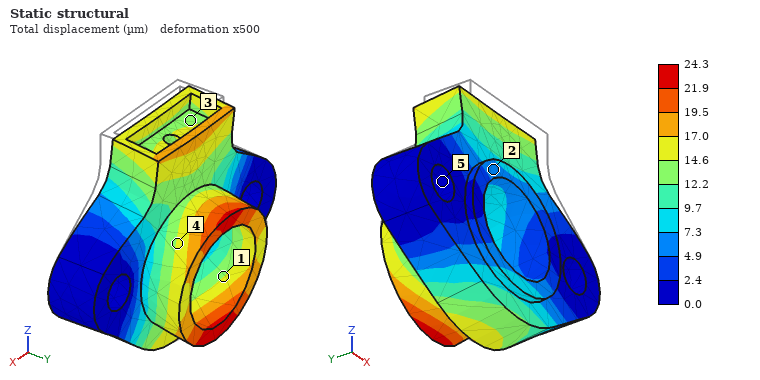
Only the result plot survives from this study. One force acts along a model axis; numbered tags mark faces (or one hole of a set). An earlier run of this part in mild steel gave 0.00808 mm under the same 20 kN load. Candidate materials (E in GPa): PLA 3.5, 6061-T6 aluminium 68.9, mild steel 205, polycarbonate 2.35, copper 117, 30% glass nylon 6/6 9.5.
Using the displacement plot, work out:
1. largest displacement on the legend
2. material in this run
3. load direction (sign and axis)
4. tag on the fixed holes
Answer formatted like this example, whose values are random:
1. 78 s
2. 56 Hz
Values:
1. 24.3 µm
2. 6061-T6 aluminium
3. -Z
4. 5
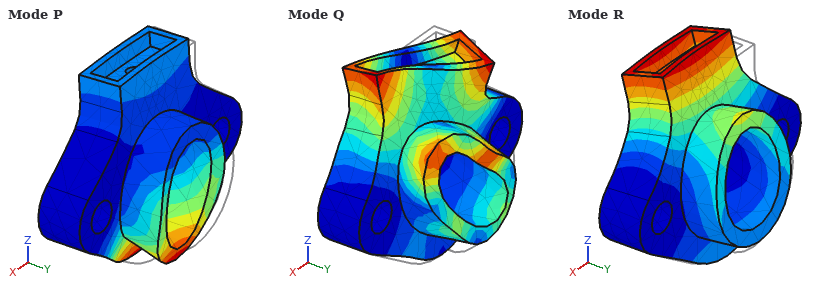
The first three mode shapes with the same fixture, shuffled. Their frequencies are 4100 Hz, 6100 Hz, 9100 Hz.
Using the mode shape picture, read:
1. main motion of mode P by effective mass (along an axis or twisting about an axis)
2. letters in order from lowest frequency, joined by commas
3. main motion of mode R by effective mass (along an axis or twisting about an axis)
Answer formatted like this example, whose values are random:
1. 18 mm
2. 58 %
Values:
1. along Y
2. R, P, Q
3. along Y
